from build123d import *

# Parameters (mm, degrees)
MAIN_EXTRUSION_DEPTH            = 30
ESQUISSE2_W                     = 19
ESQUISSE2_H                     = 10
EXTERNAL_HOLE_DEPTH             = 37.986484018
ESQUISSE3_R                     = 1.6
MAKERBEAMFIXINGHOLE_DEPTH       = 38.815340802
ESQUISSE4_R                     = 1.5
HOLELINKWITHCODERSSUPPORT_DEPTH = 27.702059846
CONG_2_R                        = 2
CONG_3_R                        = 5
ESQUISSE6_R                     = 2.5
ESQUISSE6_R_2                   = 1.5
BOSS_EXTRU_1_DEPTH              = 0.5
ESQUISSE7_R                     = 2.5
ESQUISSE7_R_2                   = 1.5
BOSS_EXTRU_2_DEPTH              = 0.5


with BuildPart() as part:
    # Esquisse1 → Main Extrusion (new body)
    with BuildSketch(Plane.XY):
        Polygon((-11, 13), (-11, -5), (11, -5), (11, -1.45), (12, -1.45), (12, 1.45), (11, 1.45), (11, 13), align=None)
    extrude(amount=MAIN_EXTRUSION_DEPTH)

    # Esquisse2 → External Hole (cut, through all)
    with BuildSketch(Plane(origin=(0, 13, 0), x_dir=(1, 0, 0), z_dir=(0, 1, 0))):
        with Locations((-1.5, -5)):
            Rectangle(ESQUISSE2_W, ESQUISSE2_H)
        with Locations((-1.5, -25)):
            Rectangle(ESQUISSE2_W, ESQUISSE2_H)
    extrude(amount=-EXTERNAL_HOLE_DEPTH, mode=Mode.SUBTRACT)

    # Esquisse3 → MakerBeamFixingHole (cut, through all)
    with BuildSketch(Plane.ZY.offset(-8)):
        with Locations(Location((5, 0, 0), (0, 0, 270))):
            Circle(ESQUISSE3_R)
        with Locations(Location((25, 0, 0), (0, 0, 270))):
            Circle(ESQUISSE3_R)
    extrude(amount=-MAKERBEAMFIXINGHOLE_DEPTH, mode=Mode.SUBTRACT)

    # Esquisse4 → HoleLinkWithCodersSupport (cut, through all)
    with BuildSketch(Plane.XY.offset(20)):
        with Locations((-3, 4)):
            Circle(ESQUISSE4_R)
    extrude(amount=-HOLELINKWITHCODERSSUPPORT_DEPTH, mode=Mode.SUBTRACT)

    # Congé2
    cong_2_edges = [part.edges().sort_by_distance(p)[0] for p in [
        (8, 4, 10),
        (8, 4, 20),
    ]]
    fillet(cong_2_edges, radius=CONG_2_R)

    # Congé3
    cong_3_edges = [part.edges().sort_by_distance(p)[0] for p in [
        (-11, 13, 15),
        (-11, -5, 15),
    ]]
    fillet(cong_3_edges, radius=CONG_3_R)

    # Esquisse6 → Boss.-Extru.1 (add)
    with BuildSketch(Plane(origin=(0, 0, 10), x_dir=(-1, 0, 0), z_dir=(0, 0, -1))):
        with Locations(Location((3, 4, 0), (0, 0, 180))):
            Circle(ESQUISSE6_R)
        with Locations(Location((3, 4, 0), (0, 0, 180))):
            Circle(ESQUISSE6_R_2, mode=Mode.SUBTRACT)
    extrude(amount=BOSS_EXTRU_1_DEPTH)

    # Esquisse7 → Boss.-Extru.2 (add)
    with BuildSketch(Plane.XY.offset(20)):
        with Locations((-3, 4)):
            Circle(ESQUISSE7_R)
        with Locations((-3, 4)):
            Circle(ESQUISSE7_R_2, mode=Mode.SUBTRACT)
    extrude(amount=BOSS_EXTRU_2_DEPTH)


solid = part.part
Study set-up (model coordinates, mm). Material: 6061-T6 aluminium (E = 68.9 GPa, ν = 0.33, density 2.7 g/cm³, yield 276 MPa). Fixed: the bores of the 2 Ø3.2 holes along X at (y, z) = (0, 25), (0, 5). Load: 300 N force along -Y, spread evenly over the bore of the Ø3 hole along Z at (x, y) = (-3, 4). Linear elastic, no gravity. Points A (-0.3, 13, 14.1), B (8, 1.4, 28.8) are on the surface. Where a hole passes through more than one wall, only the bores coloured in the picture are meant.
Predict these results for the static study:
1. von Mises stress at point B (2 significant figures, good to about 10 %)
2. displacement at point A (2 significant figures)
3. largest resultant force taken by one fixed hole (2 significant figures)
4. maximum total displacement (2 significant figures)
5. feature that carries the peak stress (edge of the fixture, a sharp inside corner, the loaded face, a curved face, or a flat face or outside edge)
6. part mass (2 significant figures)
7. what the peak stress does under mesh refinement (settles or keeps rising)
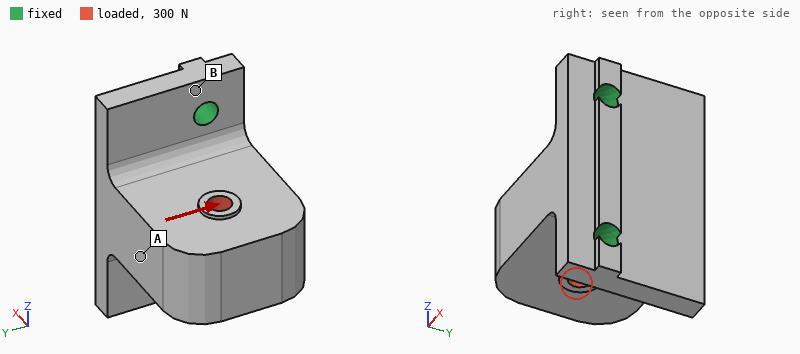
27 MPa
36 µm
160 N
50 µm
edge of the fixture
13 g
keeps rising
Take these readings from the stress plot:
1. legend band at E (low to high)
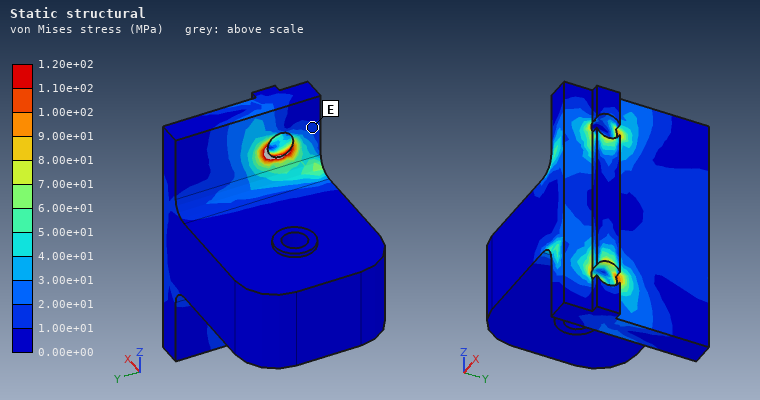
1.00e+01 to 2.00e+01 MPa
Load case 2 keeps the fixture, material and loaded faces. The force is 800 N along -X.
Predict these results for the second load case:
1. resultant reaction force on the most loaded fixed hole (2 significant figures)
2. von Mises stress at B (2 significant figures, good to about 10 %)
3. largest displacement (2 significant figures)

430 N
25 MPa
39 µm
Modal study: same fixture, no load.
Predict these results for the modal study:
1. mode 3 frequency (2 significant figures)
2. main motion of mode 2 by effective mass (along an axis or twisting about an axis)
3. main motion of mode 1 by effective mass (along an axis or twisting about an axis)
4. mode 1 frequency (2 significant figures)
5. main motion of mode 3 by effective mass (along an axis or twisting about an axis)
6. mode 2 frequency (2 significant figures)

20 kHz
along Z
along Y
4900 Hz
along X
11 kHz
